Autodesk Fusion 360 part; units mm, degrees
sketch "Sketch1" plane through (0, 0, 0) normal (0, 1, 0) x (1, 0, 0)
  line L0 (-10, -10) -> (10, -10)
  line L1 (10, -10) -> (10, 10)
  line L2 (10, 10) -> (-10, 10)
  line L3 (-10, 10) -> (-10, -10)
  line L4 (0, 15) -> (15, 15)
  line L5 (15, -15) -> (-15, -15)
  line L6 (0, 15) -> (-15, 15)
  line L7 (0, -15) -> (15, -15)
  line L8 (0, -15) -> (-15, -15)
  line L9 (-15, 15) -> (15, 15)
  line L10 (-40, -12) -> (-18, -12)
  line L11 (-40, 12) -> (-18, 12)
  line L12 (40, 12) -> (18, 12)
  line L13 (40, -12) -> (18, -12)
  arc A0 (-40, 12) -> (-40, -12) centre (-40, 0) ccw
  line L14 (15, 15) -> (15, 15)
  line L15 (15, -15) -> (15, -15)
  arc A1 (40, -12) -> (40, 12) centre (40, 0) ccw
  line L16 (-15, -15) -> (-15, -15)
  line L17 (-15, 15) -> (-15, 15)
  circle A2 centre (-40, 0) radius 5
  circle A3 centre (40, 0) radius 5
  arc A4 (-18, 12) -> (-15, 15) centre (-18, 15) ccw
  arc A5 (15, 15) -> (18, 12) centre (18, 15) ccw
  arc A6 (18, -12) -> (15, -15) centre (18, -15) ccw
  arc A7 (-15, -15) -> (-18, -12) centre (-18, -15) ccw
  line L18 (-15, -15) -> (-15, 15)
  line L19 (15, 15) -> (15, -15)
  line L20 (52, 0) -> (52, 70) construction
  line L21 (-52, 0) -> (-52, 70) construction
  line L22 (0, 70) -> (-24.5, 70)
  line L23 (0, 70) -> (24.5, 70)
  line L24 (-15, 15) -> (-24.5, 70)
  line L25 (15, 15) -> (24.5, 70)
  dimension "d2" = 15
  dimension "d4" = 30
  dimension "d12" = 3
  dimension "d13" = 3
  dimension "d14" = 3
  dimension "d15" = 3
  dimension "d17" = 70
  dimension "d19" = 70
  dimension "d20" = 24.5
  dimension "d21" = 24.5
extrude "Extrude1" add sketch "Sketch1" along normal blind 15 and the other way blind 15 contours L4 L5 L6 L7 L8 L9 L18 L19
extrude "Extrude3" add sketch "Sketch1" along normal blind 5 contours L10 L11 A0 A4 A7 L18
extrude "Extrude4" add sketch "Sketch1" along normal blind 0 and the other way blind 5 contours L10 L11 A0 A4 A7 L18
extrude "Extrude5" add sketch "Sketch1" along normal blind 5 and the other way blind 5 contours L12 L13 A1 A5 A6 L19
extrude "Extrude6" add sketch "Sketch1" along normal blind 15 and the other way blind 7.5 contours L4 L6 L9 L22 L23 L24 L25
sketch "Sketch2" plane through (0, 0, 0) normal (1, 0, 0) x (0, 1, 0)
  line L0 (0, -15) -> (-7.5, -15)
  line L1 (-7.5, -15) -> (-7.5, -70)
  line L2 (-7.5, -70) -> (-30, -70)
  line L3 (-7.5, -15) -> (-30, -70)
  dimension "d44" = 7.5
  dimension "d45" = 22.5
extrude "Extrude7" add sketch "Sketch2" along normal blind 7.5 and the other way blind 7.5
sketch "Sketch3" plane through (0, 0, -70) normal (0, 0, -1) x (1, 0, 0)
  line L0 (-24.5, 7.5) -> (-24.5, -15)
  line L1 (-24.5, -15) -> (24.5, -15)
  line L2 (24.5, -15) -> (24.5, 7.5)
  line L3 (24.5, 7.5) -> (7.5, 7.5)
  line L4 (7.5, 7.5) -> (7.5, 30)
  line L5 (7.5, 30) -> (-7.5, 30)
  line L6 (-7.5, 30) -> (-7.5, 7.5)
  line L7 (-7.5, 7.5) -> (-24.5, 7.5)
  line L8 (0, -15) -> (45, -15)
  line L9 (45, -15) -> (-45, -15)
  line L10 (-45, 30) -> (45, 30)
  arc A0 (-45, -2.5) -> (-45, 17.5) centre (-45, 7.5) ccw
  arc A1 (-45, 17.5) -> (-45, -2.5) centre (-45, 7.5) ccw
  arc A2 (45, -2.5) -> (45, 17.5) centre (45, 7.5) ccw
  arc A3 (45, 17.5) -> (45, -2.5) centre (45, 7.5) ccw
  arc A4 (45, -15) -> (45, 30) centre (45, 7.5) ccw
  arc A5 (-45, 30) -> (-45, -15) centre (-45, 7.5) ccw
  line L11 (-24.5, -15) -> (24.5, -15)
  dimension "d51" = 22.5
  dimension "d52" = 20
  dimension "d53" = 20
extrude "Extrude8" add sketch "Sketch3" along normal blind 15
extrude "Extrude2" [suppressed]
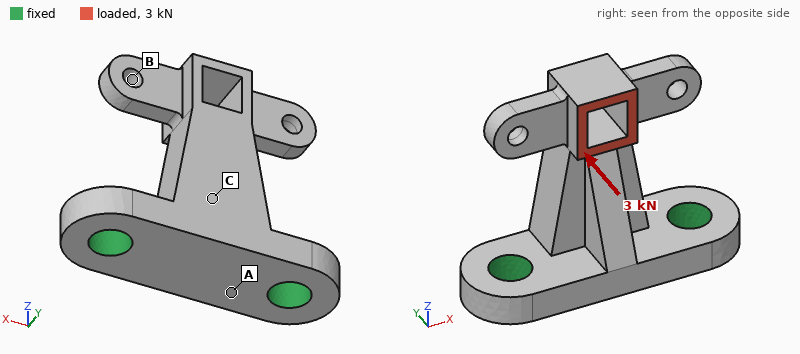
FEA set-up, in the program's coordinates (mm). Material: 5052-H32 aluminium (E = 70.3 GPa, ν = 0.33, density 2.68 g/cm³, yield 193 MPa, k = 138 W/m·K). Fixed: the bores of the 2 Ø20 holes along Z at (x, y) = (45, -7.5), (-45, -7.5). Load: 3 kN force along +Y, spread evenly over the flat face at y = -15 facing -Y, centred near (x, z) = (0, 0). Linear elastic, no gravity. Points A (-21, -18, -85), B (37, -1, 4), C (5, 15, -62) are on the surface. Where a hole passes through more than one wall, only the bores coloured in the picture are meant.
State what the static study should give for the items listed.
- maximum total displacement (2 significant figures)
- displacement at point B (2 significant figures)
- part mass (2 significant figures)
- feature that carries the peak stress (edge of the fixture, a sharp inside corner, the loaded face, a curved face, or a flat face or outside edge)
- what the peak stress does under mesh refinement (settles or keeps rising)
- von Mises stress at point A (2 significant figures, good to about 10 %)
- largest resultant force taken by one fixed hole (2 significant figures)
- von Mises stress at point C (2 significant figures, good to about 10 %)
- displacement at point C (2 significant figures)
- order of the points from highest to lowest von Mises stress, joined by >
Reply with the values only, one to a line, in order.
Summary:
0.29 mm
0.24 mm
440 g
edge of the fixture
keeps rising
28 MPa
1.5 kN
18 MPa
0.055 mm
A > C > B
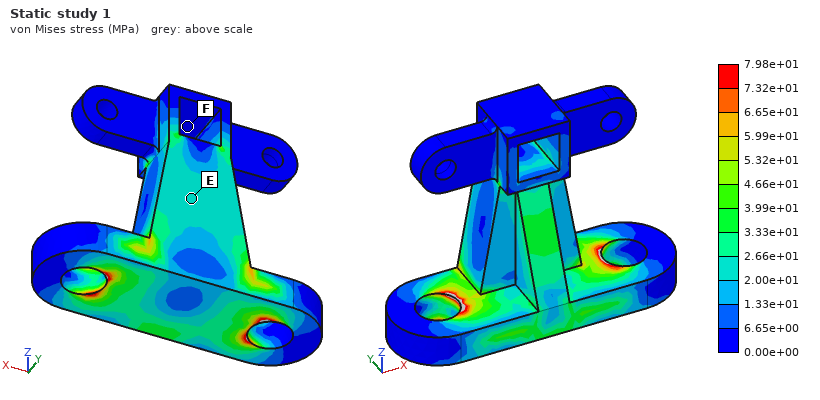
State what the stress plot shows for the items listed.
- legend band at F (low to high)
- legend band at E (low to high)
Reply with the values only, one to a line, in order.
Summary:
0.00e+00 to 6.65e+00 MPa
2.00e+01 to 2.66e+01 MPa
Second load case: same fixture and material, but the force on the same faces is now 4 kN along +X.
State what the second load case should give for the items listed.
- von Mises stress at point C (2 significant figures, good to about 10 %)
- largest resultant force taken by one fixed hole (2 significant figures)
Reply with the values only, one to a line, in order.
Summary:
18 MPa
5.4 kN
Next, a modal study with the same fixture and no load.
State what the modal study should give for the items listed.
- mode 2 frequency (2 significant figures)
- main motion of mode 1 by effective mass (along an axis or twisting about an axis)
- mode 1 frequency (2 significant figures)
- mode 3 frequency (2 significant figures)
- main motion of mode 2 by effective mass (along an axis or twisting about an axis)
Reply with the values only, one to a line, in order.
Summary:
2400 Hz
along Y
1700 Hz
3300 Hz
along X
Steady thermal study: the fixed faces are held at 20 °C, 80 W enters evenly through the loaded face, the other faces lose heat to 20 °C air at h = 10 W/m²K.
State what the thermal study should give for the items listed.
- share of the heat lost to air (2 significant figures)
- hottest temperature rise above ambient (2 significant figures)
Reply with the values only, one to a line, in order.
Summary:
10 %
76 K
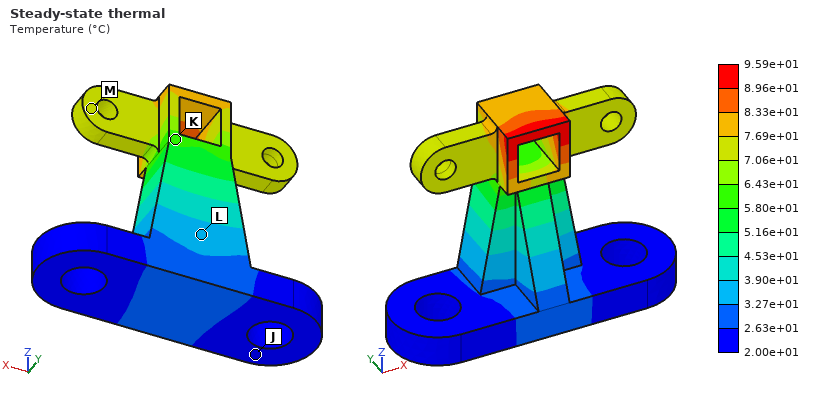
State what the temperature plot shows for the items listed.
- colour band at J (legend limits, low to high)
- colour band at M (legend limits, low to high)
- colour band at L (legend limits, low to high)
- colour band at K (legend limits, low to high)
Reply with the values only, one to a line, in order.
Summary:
2.00e+01 to 2.63e+01 °C
7.06e+01 to 7.69e+01 °C
3.27e+01 to 3.90e+01 °C
5.80e+01 to 6.43e+01 °C
